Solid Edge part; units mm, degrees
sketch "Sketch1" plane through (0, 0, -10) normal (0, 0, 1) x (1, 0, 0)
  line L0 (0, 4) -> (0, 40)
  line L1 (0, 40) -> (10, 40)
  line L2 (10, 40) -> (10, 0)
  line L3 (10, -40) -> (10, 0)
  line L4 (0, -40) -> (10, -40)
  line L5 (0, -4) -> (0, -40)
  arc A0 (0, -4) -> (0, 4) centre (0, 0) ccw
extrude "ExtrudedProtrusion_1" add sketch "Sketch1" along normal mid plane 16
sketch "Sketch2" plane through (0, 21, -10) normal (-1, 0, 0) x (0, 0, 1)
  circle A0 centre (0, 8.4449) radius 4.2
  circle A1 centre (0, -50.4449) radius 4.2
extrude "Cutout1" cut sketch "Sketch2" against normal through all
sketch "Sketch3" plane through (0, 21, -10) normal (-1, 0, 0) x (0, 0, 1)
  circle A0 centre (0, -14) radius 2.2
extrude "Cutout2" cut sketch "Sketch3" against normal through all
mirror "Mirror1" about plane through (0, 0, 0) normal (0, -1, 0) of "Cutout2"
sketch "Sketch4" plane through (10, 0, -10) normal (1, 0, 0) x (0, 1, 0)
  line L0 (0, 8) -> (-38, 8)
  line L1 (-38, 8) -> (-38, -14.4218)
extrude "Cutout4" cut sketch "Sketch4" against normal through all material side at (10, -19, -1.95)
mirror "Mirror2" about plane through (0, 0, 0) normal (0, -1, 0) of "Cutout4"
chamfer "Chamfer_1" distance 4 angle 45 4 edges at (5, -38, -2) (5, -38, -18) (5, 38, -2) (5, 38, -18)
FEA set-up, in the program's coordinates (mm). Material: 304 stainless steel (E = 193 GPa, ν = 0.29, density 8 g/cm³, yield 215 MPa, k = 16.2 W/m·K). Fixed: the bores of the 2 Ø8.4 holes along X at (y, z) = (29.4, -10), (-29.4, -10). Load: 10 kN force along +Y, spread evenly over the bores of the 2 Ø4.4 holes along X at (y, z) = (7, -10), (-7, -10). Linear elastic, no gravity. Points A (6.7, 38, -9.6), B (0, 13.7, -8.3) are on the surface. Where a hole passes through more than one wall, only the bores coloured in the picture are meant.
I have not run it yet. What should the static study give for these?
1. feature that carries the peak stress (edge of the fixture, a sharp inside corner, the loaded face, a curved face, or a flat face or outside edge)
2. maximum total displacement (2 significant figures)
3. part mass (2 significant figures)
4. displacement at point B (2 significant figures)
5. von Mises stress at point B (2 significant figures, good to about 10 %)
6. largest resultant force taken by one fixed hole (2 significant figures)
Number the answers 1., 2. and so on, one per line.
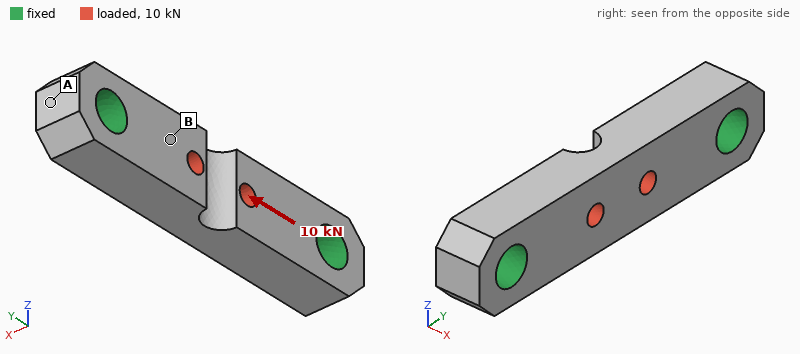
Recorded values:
1. a curved face
2. 6.6 µm
3. 80 g
4. 2.3 µm
5. 38 MPa
6. 5.0 kN
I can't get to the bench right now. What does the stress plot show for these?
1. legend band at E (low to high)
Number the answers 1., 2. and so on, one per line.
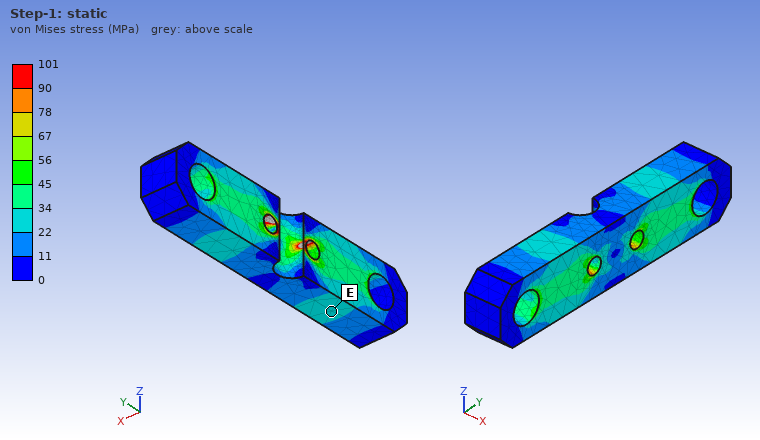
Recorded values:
1. 22 to 34 MPa
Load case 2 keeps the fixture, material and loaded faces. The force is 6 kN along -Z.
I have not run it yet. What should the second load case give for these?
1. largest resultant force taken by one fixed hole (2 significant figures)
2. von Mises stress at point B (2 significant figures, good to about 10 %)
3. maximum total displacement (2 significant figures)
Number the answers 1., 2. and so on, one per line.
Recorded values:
1. 3.0 kN
2. 46 MPa
3. 18 µm
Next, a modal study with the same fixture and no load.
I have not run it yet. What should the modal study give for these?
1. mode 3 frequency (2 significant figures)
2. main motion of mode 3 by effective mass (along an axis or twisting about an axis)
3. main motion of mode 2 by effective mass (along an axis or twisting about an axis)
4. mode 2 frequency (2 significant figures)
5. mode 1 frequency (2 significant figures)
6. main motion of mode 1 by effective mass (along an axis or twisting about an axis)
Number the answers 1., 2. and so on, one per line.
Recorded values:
1. 25 kHz
2. twisting about Y
3. along Z
4. 18 kHz
5. 14 kHz
6. along X
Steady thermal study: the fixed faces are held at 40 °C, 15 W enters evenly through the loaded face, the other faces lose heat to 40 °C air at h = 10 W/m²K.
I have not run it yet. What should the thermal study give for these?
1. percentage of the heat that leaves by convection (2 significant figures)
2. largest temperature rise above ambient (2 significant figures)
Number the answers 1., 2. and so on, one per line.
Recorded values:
1. 6.3 %
2. 66 K
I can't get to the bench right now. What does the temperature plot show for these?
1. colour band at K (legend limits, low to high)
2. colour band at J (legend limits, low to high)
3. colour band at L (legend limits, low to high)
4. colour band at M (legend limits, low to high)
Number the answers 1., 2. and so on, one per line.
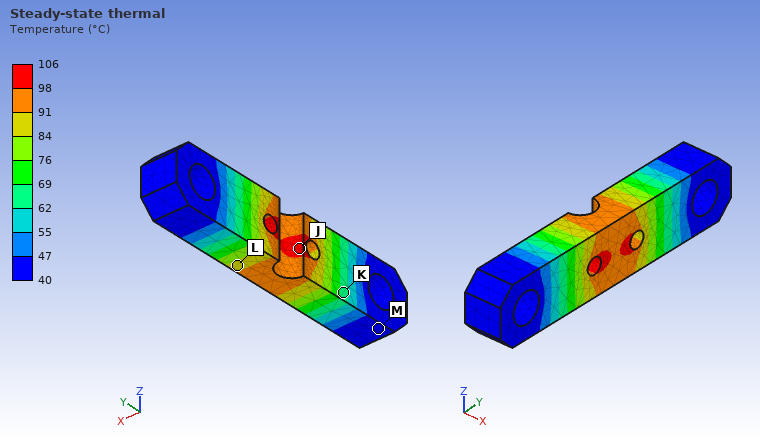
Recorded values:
1. 62 to 69 °C
2. 98 to 106 °C
3. 84 to 91 °C
4. 40 to 47 °C
